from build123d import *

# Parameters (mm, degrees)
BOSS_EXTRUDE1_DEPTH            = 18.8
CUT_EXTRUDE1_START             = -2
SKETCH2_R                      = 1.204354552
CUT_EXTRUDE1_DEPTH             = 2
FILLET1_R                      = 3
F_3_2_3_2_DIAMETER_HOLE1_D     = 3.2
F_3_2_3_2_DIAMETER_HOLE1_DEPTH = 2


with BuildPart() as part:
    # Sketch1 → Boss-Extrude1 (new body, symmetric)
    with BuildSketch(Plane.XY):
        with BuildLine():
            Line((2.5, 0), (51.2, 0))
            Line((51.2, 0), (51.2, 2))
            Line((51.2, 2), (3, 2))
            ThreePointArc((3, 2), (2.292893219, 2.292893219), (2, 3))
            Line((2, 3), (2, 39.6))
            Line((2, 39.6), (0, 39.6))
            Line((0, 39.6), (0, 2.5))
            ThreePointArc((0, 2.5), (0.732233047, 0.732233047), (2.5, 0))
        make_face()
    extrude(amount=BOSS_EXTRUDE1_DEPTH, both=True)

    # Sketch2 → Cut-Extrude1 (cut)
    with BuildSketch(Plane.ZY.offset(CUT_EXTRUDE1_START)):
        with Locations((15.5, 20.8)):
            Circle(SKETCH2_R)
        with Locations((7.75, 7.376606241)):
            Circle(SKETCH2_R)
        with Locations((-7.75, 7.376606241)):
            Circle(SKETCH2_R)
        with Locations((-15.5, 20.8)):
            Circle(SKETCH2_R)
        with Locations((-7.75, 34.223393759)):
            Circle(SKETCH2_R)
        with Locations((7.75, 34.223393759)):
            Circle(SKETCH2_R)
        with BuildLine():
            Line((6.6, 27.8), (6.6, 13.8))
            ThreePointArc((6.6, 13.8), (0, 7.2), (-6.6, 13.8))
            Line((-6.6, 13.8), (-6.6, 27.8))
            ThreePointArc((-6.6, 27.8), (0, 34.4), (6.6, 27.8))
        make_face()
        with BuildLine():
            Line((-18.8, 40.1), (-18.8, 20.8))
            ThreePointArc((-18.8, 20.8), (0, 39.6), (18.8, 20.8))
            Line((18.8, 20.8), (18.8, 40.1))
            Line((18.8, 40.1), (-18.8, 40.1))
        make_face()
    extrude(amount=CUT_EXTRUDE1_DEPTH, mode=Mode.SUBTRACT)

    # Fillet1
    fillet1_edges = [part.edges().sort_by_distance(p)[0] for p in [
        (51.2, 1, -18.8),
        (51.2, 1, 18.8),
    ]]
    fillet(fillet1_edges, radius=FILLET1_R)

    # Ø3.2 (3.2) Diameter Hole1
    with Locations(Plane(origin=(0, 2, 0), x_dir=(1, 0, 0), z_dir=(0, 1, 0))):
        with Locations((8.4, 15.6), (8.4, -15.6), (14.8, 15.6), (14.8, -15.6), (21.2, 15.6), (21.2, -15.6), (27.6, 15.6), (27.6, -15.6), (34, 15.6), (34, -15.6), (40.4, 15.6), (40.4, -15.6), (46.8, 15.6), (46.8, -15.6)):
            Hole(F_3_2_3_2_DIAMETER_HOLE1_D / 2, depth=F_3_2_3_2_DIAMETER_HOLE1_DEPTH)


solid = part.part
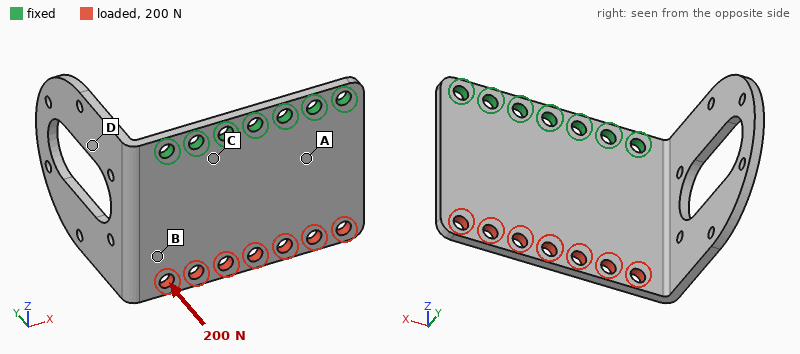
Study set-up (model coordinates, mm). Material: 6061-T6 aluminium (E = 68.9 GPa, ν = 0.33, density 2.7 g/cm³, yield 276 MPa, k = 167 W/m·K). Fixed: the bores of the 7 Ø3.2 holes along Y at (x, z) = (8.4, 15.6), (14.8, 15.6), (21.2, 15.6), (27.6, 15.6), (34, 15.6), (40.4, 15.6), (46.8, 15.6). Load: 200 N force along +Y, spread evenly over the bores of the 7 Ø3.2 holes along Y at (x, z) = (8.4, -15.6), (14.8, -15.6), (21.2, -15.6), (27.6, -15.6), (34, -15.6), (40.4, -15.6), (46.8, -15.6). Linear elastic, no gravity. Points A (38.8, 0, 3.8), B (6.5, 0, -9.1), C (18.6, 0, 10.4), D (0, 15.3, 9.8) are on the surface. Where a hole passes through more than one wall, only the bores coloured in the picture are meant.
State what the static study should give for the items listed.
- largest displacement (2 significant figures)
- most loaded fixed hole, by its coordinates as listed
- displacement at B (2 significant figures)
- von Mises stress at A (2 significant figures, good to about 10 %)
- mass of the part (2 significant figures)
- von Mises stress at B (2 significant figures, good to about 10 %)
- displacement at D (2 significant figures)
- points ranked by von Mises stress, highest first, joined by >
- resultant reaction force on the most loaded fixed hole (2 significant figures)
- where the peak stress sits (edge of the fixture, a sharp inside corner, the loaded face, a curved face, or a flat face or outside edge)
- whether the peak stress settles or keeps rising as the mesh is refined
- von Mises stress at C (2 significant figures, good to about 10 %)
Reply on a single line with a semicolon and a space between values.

0.74 mm; (8.4, 15.6); 0.29 mm; 86 MPa; 15 g; 61 MPa; 0.17 mm; C > A > B > D; 50 N; edge of the fixture; keeps rising; 110 MPa
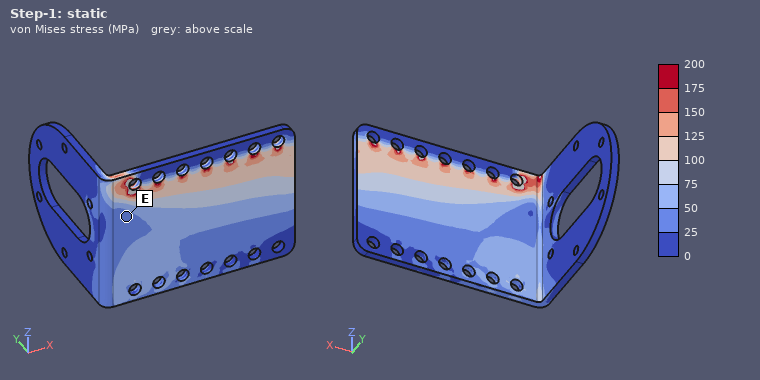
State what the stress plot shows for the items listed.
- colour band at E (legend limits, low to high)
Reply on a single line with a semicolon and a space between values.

25 to 50 MPa
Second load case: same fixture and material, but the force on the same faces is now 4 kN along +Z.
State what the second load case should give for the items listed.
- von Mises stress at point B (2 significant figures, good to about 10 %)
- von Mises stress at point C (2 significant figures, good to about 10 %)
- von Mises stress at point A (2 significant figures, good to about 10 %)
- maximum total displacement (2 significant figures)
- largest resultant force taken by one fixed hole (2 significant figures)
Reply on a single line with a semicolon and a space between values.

29 MPa; 37 MPa; 44 MPa; 22 µm; 760 N
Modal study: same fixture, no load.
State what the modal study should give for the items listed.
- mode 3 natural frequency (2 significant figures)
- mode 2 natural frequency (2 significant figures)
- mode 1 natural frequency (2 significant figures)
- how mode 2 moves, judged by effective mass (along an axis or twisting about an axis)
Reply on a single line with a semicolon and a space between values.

2200 Hz; 1200 Hz; 900 Hz; along Y
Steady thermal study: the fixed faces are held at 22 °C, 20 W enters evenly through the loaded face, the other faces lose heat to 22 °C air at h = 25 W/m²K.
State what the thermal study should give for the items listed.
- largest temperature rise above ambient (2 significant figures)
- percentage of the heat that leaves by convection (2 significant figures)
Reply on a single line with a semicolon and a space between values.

37 K; 11 %
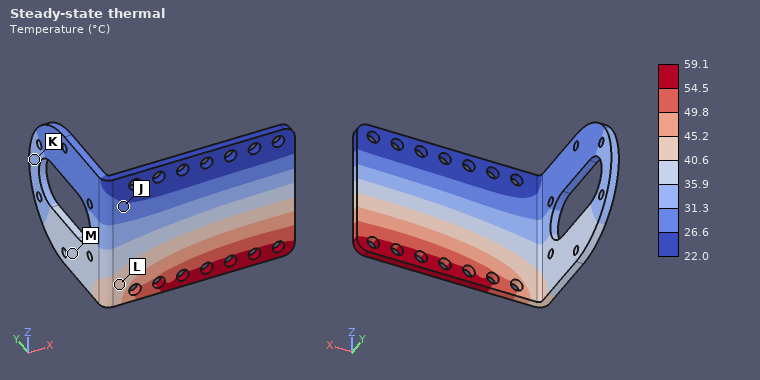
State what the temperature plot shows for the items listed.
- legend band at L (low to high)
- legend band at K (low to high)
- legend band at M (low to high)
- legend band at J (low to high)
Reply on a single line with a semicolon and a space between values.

40.6 to 45.2 °C; 31.3 to 35.9 °C; 35.9 to 40.6 °C; 26.6 to 31.3 °C
